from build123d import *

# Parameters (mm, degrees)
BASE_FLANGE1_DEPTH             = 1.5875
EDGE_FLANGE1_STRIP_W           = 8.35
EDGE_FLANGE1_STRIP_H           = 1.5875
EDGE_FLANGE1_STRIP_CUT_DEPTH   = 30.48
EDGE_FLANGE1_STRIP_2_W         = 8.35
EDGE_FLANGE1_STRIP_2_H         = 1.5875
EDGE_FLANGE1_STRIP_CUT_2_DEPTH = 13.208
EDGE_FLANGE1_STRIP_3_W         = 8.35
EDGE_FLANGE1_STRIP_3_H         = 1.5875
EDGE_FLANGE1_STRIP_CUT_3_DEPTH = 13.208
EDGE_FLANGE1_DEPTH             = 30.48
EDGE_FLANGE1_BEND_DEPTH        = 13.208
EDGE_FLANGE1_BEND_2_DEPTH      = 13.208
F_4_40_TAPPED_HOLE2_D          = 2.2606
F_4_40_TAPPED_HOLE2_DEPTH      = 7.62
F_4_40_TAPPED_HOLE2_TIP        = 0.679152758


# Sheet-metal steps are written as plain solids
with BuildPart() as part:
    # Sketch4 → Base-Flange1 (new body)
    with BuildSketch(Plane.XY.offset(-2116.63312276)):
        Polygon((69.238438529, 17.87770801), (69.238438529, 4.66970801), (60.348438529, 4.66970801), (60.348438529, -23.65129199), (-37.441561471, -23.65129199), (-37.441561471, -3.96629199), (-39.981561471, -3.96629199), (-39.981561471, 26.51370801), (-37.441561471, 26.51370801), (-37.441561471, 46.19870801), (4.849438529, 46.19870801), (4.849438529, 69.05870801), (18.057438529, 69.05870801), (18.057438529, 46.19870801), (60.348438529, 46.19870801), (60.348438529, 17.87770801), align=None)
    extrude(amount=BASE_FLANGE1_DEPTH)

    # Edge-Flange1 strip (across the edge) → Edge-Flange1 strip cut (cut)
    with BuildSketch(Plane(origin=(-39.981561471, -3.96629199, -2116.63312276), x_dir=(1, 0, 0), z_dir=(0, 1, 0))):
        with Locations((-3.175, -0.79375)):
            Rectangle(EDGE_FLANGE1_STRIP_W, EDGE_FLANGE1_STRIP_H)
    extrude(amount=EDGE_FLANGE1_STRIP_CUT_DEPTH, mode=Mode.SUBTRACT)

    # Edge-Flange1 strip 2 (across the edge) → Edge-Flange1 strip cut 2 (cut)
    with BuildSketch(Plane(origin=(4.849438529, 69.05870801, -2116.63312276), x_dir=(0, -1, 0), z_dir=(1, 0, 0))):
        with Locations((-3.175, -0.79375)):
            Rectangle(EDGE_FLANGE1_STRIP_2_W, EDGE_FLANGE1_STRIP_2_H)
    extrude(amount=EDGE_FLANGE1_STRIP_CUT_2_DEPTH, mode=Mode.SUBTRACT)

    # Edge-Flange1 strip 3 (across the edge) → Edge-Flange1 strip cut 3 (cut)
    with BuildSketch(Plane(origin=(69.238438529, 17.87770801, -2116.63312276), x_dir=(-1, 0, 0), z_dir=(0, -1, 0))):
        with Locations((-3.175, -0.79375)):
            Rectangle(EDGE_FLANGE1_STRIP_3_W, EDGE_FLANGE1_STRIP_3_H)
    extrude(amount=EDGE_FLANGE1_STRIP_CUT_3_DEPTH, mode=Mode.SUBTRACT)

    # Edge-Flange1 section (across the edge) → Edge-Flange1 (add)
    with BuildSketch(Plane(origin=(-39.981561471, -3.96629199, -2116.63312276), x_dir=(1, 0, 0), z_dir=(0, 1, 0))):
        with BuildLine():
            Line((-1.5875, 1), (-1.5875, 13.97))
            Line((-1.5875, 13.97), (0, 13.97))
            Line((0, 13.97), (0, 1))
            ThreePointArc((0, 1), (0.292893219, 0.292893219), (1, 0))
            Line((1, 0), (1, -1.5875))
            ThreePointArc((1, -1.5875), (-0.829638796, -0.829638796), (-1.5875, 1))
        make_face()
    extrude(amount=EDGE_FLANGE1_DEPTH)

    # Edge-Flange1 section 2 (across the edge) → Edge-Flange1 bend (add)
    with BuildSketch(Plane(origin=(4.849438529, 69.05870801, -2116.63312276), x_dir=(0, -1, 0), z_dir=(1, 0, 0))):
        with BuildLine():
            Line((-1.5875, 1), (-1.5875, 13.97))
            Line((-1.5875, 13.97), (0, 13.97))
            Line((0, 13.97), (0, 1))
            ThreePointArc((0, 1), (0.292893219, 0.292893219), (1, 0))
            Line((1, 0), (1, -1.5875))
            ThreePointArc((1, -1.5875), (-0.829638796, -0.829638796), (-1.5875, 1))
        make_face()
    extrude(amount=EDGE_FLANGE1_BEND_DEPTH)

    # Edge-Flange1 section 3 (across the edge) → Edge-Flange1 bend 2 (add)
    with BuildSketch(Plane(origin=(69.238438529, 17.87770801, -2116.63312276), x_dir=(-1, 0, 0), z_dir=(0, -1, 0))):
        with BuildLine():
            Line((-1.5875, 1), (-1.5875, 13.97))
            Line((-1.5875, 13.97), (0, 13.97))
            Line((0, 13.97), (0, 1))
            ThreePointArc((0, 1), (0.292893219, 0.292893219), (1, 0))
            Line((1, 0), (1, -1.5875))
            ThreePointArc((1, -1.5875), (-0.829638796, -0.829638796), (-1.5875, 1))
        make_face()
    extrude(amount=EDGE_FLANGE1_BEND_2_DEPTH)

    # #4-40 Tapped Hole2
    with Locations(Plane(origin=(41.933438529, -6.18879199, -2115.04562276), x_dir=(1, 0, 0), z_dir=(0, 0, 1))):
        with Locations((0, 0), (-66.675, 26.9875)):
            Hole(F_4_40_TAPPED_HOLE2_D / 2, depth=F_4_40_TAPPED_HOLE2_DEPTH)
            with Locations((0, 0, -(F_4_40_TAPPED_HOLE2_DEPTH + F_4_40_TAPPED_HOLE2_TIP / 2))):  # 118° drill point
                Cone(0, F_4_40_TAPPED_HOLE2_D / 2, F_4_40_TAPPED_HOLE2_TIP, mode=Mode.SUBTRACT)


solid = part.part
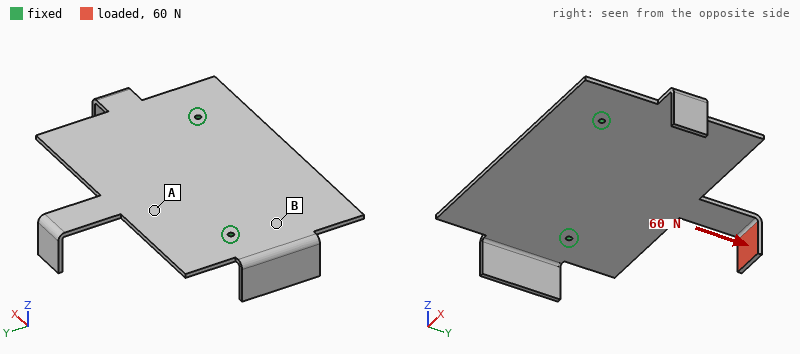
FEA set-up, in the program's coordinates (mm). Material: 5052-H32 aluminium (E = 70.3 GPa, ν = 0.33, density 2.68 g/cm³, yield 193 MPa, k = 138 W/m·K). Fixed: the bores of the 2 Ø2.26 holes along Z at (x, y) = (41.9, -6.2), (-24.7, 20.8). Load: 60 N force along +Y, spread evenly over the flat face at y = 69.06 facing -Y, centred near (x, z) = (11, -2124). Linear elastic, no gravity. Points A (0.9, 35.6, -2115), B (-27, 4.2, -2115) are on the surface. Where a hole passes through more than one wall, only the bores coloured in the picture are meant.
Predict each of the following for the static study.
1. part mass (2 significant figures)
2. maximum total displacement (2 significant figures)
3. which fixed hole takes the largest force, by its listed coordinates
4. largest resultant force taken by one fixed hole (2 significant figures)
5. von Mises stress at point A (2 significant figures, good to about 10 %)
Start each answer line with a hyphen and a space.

- 35 g
- 1.5 mm
- (41.9, -6.2)
- 35 N
- 22 MPa
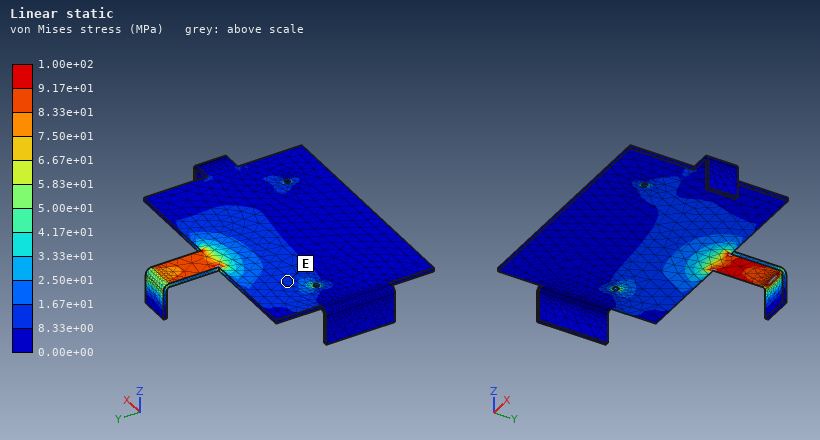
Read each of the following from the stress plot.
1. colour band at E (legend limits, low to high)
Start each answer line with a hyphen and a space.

- 8.33e+00 to 1.67e+01 MPa
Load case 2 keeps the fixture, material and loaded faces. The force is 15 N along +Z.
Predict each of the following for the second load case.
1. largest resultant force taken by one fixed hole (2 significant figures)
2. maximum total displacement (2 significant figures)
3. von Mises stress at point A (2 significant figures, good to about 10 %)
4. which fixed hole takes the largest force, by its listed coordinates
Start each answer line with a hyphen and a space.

- 12 N
- 1.3 mm
- 26 MPa
- (-24.7, 20.8)
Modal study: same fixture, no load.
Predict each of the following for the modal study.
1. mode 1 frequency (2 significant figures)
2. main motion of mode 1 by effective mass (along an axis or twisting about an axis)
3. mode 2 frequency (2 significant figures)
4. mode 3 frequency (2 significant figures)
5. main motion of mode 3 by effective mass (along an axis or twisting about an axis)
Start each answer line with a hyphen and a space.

- 380 Hz
- along Z
- 720 Hz
- 800 Hz
- along Z
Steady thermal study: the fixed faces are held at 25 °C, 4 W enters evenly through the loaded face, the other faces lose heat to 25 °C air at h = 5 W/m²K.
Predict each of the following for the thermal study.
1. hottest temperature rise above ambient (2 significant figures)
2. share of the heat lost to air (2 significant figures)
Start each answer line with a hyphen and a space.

- 60 K
- 14 %
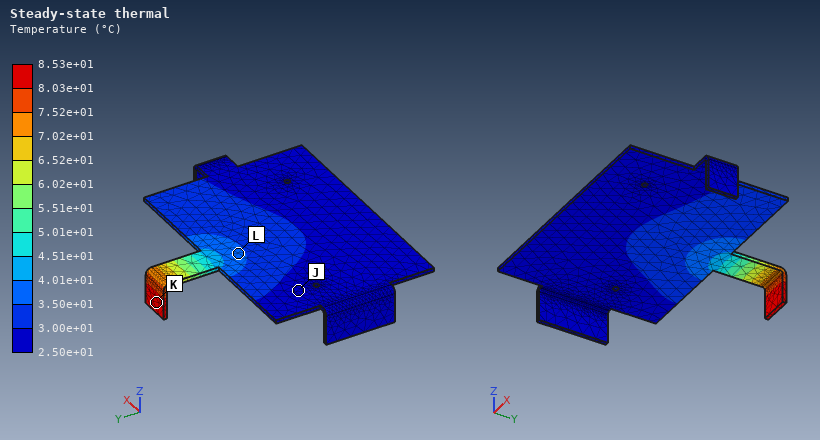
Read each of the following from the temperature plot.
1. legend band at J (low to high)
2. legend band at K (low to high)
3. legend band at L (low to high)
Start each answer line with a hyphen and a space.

- 2.50e+01 to 3.00e+01 °C
- 8.03e+01 to 8.53e+01 °C
- 3.50e+01 to 4.01e+01 °C
